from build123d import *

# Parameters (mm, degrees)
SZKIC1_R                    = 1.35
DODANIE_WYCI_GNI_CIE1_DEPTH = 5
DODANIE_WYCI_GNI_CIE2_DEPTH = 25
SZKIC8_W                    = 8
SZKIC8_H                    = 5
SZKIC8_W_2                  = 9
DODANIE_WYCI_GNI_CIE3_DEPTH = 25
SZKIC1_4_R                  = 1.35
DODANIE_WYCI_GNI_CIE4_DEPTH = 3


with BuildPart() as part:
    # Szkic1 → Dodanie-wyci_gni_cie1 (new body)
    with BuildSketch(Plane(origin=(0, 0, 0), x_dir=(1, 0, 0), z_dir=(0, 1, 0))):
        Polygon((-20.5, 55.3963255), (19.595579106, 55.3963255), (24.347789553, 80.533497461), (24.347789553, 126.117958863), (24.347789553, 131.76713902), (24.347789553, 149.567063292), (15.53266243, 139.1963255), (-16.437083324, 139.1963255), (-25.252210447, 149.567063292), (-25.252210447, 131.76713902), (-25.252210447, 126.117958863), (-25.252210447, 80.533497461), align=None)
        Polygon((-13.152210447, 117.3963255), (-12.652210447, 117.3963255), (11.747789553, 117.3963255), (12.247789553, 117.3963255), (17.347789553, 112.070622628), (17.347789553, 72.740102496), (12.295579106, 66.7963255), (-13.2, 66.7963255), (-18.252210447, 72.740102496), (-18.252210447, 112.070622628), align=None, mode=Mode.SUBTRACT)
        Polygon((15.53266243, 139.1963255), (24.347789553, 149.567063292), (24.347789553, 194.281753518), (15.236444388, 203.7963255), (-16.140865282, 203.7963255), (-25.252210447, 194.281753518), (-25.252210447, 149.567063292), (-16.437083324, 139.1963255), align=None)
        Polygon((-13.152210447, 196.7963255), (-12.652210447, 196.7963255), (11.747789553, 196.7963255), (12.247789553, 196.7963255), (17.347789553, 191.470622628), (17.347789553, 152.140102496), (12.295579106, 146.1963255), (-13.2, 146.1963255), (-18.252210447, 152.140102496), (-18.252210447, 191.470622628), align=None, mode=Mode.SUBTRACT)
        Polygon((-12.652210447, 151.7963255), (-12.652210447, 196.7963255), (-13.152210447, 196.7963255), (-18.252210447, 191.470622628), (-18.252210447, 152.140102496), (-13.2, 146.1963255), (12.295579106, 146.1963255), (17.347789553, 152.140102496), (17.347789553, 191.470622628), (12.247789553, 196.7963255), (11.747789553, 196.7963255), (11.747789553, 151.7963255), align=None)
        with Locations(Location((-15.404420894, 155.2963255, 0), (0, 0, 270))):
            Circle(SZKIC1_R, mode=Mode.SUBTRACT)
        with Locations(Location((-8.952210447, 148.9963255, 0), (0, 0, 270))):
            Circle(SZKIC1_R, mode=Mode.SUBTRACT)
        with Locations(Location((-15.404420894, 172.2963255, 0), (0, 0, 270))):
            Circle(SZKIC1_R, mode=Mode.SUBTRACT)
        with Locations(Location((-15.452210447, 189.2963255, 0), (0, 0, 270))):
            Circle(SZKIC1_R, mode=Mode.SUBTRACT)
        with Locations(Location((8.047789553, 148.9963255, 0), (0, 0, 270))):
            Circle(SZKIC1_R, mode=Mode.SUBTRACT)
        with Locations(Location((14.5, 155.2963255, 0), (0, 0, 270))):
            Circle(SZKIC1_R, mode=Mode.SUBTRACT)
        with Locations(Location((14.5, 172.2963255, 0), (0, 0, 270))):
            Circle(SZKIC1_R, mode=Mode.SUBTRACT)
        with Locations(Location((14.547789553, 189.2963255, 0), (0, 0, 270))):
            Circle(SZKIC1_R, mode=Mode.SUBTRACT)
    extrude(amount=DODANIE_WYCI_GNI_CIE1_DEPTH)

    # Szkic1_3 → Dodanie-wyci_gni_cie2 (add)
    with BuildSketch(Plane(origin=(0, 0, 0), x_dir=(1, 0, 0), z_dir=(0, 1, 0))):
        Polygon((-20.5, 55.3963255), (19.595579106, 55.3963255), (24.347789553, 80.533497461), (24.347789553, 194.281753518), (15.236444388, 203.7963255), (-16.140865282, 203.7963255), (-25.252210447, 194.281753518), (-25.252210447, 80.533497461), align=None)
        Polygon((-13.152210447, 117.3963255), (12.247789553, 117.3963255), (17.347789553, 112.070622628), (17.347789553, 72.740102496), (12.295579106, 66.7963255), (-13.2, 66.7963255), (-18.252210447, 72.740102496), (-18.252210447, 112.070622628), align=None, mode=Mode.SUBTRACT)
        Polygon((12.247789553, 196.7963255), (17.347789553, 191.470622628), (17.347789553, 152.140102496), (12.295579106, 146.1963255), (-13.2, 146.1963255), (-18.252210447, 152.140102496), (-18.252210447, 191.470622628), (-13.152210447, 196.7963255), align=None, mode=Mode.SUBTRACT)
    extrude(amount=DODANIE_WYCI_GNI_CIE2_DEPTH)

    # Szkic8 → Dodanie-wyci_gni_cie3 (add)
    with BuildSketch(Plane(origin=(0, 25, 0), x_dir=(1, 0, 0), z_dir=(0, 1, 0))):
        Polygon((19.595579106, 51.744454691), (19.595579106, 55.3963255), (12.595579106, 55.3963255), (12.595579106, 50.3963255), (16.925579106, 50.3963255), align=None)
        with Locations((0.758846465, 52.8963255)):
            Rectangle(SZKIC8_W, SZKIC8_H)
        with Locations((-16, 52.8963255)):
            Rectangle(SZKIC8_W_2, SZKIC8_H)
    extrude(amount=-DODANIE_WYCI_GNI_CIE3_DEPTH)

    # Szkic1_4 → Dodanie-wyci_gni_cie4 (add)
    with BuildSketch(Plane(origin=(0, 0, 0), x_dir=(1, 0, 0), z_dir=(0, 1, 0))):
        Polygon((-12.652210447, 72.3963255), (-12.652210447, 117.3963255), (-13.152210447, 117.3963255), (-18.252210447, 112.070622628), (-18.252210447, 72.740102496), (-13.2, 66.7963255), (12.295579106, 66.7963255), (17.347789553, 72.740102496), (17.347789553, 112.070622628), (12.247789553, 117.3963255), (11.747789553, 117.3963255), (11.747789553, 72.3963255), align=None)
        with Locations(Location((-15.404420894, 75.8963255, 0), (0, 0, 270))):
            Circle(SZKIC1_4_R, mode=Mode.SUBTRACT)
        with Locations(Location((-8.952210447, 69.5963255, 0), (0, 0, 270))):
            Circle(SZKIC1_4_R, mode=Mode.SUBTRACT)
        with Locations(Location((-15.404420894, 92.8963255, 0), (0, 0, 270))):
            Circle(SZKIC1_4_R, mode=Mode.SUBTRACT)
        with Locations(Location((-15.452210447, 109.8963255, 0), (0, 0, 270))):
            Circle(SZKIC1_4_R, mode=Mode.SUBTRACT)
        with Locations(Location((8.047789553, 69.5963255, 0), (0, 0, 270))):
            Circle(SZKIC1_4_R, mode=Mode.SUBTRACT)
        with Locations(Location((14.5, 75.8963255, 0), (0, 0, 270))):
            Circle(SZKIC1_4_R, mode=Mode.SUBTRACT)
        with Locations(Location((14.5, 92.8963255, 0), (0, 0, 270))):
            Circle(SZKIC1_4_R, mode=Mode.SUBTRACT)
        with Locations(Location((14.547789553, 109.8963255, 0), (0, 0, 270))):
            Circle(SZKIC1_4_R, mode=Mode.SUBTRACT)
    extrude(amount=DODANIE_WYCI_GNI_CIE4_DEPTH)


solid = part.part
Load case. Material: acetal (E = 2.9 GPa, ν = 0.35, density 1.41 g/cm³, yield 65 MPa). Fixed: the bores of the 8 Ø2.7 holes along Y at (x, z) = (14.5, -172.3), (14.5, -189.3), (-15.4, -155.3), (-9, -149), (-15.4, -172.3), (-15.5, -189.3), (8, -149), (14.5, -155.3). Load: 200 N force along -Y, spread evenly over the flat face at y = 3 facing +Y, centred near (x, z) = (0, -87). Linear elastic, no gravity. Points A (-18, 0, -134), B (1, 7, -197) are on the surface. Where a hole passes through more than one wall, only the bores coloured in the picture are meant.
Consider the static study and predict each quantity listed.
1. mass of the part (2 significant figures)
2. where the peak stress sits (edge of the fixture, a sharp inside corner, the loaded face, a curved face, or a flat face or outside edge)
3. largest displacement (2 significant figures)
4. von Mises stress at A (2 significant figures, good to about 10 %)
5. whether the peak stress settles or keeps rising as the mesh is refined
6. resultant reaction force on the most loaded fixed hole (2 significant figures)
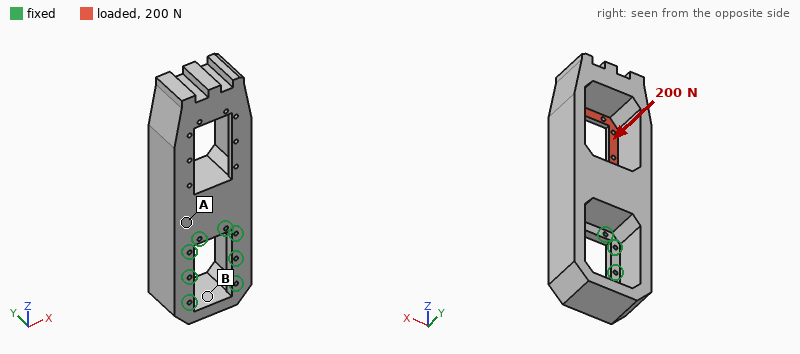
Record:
140 g
edge of the fixture
0.68 mm
2.2 MPa
keeps rising
250 N
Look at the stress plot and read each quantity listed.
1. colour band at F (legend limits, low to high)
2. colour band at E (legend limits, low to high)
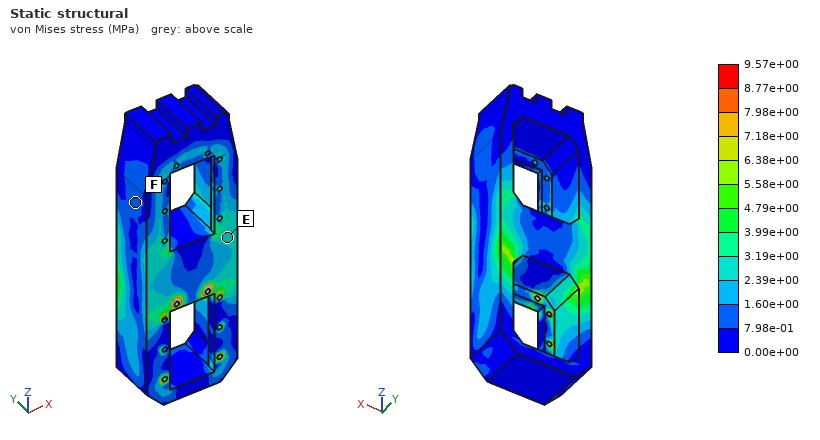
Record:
7.98e-01 to 1.60e+00 MPa
2.39e+00 to 3.19e+00 MPa
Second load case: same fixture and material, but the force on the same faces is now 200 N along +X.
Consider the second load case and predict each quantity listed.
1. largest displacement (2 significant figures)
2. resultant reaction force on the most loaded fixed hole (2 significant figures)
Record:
0.42 mm
140 N
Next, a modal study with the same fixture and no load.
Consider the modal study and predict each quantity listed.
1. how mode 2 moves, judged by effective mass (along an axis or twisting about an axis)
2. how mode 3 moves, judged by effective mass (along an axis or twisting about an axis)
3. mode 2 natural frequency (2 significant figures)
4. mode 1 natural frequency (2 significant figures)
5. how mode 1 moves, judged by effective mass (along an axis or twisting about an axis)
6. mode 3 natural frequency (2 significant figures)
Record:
along X
twisting about Z
500 Hz
400 Hz
along Y
1000 Hz
